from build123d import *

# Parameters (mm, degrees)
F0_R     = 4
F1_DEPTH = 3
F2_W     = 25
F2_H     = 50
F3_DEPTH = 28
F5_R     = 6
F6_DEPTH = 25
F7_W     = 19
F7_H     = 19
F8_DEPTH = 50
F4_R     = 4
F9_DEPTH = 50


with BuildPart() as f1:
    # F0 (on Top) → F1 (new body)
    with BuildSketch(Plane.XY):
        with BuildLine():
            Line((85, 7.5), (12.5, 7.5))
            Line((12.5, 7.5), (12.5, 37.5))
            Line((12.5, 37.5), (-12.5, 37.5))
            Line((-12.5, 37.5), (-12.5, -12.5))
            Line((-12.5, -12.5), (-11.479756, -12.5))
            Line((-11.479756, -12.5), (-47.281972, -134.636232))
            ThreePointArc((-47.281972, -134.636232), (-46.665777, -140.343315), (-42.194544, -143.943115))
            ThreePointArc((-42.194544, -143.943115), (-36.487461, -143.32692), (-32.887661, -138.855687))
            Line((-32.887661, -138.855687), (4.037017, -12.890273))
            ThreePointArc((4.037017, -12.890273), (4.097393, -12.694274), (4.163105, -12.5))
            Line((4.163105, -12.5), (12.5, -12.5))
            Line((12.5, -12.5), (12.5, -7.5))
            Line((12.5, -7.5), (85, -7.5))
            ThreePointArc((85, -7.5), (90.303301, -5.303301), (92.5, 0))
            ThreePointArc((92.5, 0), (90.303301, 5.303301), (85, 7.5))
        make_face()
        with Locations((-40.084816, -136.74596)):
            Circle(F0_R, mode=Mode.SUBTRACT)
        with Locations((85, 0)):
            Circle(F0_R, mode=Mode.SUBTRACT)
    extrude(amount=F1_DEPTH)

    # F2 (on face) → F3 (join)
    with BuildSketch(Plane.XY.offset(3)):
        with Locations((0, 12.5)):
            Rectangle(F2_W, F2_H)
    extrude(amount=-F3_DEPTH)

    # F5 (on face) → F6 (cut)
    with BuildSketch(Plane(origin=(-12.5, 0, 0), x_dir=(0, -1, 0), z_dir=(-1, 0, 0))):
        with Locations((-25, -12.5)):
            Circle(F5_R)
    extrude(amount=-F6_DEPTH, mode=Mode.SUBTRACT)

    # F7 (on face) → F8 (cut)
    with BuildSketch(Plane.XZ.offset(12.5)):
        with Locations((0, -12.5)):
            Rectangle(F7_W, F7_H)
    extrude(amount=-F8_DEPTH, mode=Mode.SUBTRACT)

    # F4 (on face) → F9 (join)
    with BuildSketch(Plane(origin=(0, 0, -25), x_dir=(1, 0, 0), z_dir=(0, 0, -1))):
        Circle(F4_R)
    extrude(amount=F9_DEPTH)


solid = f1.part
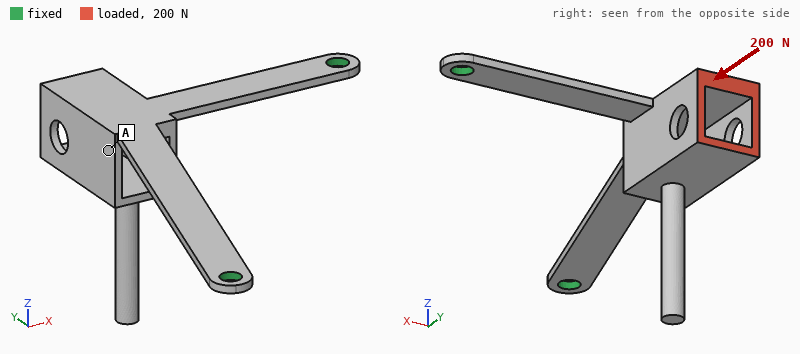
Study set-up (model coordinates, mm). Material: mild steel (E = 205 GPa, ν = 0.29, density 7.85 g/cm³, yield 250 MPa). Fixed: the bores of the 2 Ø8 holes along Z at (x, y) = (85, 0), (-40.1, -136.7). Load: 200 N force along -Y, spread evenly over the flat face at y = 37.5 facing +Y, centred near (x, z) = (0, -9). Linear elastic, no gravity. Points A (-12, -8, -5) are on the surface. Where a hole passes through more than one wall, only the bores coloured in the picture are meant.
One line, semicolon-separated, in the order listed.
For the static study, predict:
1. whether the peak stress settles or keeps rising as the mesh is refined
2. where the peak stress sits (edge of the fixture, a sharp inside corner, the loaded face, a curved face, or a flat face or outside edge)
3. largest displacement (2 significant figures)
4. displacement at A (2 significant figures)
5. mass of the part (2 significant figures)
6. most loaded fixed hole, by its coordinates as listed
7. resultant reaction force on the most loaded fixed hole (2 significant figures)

keeps rising; edge of the fixture; 0.67 mm; 0.20 mm; 220 g; (-40.1, -136.7); 200 N
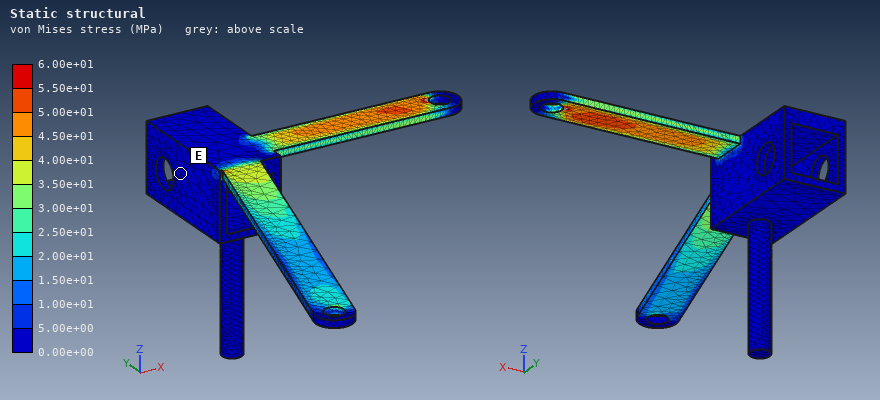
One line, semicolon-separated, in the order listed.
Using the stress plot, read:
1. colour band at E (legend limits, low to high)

0.00e+00 to 5.00e+00 MPa
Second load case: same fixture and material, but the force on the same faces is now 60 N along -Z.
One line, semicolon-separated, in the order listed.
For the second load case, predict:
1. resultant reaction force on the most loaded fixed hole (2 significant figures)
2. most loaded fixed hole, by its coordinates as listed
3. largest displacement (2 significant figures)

54 N; (85, 0); 1.7 mm
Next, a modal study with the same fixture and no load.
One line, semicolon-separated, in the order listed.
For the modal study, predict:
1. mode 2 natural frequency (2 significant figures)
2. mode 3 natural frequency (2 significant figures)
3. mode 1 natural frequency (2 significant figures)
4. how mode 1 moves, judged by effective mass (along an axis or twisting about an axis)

290 Hz; 440 Hz; 100 Hz; along Z
